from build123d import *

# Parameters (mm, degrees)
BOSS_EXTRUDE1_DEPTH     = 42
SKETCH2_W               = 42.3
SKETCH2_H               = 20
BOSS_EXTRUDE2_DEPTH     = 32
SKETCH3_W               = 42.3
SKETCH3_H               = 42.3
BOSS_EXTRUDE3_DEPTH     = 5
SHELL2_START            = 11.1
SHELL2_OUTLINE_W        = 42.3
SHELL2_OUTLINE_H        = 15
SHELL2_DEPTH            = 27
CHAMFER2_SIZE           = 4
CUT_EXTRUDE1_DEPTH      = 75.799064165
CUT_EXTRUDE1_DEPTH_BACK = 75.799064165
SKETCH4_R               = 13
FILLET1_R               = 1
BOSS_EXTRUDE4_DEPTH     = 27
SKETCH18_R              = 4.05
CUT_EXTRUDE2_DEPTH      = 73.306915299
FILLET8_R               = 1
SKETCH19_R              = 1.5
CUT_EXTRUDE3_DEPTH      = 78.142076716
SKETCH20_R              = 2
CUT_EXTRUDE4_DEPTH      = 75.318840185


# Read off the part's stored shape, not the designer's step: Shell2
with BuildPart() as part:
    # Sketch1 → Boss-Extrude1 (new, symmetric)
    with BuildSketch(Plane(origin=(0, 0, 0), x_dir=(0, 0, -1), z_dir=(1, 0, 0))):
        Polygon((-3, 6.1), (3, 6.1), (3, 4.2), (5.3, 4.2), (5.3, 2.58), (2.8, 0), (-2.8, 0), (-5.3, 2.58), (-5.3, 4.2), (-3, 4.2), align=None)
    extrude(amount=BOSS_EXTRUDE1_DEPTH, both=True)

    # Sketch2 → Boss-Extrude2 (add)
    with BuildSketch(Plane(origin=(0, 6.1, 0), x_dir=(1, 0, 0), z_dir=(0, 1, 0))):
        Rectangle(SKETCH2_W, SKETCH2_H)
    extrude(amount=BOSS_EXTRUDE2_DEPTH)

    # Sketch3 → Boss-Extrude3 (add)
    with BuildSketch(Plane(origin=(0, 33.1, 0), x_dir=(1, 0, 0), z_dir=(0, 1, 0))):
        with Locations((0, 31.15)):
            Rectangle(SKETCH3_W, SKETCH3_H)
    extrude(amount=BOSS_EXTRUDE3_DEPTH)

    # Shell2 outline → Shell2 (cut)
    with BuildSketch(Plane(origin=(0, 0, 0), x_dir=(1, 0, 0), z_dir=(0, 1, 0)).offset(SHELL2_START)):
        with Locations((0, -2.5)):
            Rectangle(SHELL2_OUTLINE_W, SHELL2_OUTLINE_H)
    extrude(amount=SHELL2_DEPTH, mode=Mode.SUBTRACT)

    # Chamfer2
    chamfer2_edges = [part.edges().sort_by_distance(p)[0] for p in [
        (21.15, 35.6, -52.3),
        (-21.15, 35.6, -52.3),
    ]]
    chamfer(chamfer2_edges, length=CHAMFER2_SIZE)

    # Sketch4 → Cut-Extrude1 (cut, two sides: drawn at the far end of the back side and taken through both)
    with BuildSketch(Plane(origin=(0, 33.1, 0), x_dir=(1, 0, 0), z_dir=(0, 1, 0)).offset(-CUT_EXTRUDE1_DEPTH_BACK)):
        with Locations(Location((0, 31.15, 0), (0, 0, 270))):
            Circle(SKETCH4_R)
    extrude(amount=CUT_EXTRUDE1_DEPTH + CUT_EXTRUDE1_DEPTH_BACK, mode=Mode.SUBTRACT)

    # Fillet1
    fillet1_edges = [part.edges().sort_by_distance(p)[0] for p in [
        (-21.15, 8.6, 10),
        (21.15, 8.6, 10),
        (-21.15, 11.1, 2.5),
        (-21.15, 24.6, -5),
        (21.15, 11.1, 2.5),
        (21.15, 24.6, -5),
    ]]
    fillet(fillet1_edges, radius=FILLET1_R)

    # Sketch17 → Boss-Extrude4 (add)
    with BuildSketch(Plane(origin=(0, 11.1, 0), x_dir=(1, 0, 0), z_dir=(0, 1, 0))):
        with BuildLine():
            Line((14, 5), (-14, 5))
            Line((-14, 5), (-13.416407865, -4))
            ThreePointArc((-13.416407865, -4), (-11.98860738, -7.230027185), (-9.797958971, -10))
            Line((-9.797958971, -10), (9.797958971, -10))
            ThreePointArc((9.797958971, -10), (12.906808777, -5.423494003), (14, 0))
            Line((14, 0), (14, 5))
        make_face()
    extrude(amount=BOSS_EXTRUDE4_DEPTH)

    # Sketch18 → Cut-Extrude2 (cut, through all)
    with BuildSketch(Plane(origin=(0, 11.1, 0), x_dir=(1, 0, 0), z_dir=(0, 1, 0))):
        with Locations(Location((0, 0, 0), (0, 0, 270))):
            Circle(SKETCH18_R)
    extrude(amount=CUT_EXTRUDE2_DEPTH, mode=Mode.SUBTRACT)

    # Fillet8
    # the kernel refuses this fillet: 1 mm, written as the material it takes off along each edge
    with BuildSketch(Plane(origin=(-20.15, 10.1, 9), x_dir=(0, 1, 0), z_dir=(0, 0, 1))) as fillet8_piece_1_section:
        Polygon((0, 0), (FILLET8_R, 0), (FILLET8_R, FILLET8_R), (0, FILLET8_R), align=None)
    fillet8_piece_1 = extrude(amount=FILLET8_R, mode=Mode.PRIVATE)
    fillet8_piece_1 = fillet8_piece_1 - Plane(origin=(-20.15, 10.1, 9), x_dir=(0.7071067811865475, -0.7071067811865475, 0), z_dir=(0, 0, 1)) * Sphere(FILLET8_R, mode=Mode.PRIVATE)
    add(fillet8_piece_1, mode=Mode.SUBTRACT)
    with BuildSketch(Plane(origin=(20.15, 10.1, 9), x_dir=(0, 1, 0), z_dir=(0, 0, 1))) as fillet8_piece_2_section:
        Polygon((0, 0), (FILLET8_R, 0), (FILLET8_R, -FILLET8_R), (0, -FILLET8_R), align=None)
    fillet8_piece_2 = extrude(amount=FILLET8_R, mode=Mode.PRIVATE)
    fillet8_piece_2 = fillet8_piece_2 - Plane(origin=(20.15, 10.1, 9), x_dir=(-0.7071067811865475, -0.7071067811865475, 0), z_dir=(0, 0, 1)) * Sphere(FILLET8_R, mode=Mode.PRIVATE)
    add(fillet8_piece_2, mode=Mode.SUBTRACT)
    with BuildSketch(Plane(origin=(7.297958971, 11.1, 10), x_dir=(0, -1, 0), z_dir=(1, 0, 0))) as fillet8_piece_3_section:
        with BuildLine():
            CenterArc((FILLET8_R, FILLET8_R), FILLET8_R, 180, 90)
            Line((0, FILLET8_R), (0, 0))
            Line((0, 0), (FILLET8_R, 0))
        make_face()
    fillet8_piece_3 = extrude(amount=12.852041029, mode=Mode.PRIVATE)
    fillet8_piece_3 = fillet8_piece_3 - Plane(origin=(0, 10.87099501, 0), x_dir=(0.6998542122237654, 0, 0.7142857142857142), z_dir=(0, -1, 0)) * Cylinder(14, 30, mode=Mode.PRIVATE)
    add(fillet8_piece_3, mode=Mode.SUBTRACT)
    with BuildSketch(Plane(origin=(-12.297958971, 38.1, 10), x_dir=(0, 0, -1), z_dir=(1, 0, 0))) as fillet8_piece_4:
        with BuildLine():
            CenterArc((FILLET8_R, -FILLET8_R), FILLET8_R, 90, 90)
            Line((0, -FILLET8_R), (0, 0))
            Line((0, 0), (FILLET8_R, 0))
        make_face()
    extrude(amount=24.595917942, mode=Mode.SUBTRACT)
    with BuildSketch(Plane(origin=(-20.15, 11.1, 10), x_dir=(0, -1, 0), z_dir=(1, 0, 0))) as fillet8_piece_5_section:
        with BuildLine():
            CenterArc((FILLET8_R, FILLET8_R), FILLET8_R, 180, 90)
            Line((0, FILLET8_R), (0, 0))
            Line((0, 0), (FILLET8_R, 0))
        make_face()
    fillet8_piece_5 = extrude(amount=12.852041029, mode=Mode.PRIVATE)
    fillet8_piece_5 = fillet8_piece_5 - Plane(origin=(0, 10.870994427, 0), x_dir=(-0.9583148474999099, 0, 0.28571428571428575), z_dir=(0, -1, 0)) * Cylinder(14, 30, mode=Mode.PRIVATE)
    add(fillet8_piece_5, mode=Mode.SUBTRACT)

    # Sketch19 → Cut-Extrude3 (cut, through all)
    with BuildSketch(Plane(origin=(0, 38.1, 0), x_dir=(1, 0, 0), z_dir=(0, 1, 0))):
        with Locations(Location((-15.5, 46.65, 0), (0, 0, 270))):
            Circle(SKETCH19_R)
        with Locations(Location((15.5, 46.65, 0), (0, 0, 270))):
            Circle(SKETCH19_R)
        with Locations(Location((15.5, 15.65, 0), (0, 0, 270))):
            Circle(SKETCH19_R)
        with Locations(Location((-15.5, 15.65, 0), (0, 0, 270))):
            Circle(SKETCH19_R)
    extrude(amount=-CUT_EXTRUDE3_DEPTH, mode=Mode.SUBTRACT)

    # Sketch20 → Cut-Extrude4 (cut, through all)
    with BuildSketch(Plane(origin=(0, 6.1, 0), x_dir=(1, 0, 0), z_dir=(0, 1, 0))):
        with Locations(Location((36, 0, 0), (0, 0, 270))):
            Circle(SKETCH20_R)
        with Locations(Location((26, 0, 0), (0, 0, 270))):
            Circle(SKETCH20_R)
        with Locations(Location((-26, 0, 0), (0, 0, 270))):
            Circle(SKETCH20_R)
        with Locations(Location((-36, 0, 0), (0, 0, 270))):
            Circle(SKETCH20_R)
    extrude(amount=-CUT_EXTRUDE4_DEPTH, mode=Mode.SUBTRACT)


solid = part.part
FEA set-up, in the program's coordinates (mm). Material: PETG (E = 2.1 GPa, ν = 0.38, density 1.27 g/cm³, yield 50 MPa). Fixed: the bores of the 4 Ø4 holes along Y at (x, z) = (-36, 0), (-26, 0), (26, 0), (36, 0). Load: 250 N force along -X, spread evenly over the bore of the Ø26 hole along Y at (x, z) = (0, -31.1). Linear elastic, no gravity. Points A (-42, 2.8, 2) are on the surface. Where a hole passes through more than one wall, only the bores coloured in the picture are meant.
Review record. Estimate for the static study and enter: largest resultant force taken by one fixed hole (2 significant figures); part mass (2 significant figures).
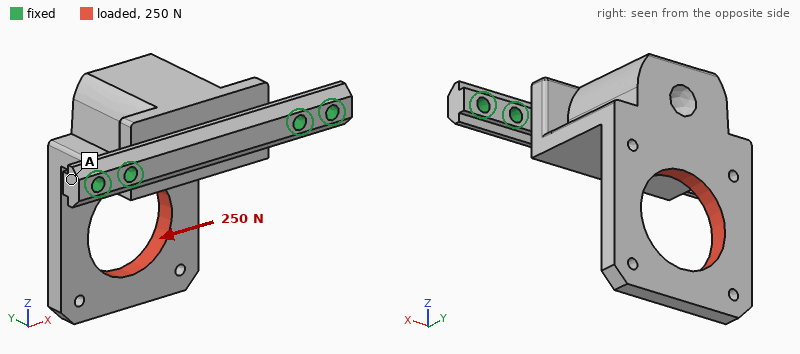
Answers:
290 N
37 g
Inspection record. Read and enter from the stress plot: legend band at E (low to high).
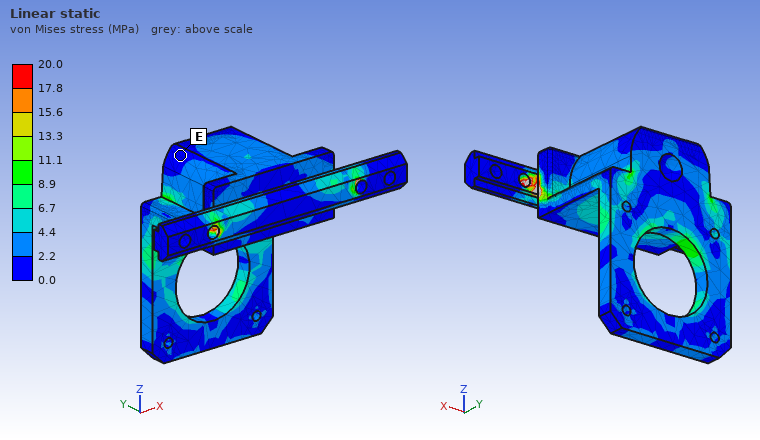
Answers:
0.0 to 2.2 MPa
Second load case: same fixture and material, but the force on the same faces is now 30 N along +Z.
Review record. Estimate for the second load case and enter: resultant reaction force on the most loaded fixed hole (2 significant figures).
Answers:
15 N
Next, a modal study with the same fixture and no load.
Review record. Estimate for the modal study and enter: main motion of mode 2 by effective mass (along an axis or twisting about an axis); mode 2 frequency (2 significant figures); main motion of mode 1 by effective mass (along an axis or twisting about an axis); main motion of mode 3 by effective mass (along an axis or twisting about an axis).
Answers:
along Z
560 Hz
along Z
along X
